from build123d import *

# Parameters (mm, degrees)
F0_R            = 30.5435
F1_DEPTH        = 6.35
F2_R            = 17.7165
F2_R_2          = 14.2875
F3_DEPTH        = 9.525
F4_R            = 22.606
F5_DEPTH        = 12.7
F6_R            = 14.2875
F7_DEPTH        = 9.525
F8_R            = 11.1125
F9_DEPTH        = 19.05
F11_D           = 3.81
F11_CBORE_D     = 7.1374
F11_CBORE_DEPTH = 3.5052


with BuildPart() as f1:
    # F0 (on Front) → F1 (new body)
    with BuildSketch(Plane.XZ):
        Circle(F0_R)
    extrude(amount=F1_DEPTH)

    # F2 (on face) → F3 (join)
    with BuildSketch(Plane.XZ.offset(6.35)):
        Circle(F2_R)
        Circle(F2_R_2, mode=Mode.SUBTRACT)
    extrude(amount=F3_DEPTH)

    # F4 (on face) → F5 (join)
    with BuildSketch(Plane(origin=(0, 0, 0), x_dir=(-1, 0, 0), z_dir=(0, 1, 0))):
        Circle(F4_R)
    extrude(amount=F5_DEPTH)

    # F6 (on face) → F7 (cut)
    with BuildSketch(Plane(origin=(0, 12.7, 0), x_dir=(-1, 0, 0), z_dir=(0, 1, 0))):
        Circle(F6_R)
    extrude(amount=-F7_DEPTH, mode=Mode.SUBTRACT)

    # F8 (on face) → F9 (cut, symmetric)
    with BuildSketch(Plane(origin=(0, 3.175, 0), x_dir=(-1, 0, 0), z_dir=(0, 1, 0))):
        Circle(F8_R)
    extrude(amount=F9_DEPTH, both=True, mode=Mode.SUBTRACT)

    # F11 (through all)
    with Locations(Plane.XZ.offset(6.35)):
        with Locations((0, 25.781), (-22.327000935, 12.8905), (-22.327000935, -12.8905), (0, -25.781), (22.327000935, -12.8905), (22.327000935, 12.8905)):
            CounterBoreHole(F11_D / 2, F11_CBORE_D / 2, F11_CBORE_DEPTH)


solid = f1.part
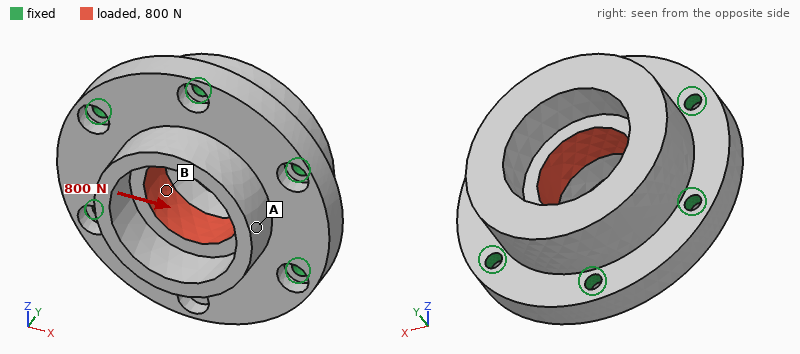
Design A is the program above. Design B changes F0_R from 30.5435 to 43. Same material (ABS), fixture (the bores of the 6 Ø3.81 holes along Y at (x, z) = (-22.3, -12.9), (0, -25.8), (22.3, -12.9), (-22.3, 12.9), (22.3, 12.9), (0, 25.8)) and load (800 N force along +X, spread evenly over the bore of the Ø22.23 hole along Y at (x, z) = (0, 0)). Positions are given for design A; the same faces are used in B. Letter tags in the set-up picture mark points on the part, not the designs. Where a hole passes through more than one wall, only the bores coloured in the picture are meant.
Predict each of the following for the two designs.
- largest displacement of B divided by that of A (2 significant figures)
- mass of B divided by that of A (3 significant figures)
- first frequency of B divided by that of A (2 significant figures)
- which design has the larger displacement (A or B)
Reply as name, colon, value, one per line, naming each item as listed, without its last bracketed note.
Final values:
largest displacement of B divided by that of A: 0.91
mass of B divided by that of A: 1.58
first frequency of B divided by that of A: 0.56
which design has the larger displacement: A
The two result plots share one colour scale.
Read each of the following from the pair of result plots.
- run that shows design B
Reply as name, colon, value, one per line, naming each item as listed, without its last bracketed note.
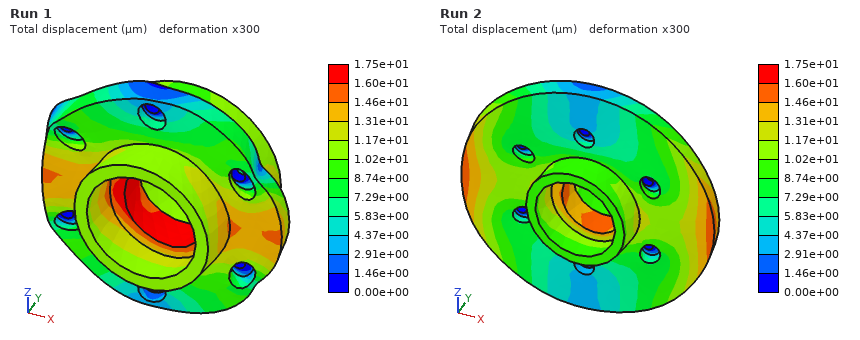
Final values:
run that shows design B: Run 2
